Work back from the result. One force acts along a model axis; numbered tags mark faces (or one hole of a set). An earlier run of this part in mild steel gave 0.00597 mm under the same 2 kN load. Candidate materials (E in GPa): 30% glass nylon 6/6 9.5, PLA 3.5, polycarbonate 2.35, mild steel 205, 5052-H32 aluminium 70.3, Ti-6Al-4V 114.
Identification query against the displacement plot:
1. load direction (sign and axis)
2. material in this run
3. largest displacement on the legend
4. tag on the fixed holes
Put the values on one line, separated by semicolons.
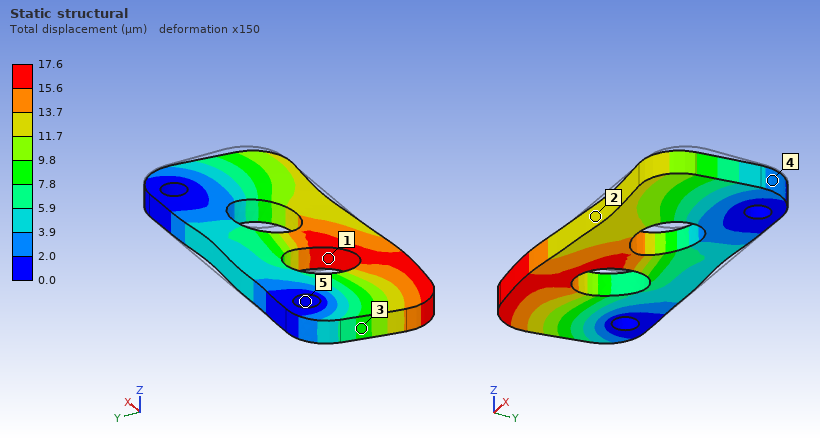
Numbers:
-X; 5052-H32 aluminium; 17.6 µm; 5
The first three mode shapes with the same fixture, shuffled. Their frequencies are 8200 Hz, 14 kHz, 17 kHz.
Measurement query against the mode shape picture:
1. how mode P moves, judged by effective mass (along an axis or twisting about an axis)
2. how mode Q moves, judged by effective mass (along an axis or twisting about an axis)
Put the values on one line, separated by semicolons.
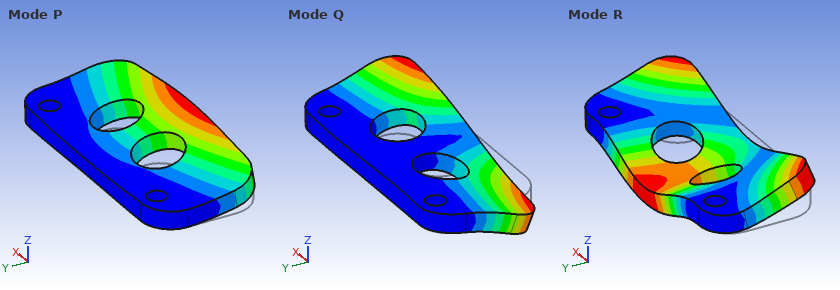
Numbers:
along Z; twisting about Y
